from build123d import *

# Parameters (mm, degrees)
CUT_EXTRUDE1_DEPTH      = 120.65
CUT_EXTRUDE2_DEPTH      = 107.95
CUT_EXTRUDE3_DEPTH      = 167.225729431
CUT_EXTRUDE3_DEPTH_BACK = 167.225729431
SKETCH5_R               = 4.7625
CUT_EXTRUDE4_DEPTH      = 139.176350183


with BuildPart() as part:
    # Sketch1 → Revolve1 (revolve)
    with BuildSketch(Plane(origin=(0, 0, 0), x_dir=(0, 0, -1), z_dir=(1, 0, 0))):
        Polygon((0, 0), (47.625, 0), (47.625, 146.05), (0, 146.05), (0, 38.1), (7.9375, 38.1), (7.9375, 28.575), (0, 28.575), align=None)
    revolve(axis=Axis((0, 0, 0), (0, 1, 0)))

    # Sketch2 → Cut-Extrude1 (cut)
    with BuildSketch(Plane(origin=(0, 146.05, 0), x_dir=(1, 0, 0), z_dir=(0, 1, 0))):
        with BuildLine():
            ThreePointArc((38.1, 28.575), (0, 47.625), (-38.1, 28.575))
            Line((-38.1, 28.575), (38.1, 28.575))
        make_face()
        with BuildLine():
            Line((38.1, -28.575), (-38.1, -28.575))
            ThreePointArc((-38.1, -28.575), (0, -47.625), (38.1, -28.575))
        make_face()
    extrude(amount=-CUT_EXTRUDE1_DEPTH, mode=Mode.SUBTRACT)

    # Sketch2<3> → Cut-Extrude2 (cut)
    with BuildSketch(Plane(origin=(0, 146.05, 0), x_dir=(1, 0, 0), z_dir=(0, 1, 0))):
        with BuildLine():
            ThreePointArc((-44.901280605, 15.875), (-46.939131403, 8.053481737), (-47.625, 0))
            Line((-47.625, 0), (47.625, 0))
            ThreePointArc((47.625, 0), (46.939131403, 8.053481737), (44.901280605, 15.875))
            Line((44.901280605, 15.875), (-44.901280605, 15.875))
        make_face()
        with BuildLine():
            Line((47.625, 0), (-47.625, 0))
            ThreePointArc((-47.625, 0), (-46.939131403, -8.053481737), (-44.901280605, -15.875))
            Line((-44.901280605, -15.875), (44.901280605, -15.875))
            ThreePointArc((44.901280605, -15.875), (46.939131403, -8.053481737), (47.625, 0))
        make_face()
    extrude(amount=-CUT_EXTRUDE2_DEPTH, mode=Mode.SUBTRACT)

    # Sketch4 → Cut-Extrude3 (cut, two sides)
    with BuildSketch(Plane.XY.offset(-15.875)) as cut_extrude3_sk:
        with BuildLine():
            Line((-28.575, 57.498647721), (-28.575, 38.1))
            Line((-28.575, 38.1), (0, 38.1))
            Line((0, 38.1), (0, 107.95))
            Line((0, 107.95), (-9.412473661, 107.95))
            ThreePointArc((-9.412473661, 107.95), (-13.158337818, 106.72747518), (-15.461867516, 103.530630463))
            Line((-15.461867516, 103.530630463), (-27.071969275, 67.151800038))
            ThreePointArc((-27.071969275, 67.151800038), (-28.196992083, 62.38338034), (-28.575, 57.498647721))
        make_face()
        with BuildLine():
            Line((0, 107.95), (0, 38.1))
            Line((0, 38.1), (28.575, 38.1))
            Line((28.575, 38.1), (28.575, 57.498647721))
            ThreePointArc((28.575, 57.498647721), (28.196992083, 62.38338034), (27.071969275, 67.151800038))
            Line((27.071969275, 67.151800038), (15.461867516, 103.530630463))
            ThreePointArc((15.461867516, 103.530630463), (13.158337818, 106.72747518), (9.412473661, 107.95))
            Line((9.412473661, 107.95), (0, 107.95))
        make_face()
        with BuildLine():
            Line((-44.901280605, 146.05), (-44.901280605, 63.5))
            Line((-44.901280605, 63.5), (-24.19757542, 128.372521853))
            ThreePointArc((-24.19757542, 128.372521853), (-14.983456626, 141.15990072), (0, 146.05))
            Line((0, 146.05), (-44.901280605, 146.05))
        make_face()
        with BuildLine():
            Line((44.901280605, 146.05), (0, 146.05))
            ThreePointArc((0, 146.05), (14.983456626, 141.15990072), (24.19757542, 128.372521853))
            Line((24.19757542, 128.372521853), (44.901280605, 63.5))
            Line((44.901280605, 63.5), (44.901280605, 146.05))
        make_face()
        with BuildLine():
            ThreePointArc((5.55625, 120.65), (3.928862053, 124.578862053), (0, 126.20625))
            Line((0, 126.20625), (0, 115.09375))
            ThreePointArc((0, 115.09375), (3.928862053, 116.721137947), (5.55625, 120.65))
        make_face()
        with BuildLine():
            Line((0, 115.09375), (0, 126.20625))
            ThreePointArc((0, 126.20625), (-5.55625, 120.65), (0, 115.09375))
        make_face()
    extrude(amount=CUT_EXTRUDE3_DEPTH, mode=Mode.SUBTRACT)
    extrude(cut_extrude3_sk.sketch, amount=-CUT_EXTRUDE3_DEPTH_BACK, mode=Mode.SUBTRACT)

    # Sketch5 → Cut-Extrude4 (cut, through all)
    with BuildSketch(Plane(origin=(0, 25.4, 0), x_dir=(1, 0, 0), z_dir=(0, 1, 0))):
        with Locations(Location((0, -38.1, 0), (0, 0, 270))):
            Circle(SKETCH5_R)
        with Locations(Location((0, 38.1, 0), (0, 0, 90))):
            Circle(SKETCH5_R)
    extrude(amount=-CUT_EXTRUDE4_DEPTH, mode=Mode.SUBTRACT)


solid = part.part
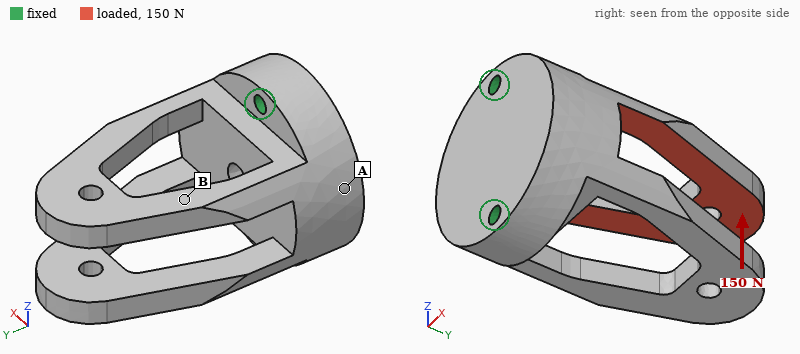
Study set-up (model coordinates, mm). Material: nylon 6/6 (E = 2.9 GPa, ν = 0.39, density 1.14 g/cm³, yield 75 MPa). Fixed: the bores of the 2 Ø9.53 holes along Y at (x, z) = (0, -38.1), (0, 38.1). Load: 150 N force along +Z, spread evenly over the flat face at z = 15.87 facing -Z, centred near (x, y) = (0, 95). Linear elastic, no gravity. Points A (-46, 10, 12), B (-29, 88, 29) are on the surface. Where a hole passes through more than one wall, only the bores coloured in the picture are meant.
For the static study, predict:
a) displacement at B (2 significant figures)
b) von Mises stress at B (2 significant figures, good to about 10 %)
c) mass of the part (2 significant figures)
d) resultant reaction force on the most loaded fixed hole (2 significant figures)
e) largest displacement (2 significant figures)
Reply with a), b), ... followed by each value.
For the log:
a) 0.85 mm
b) 3.1 MPa
c) 380 g
d) 190 N
e) 2.4 mm
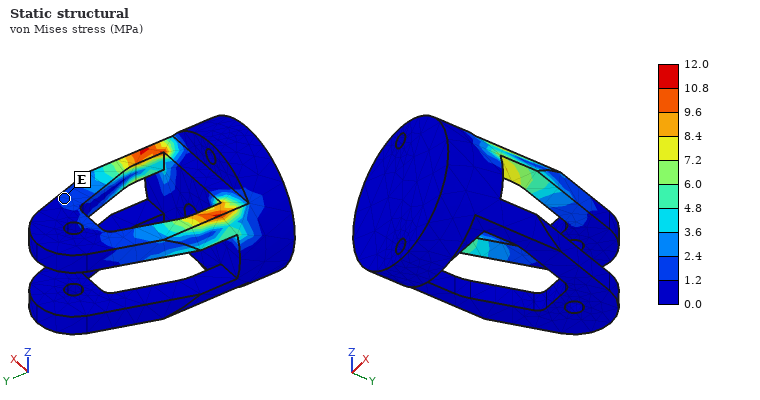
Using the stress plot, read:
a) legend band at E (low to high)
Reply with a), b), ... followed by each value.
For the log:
a) 1.2 to 2.4 MPa
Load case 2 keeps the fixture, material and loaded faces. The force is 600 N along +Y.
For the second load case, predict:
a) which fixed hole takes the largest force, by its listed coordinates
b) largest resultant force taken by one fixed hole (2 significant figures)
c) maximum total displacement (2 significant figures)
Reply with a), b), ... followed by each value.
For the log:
a) (0, 38.1)
b) 440 N
c) 1.2 mm
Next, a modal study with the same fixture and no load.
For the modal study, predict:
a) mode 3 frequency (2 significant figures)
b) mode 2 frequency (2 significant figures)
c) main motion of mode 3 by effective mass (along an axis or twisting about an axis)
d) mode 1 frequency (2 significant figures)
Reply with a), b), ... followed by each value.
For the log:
a) 480 Hz
b) 210 Hz
c) along X
d) 210 Hz
